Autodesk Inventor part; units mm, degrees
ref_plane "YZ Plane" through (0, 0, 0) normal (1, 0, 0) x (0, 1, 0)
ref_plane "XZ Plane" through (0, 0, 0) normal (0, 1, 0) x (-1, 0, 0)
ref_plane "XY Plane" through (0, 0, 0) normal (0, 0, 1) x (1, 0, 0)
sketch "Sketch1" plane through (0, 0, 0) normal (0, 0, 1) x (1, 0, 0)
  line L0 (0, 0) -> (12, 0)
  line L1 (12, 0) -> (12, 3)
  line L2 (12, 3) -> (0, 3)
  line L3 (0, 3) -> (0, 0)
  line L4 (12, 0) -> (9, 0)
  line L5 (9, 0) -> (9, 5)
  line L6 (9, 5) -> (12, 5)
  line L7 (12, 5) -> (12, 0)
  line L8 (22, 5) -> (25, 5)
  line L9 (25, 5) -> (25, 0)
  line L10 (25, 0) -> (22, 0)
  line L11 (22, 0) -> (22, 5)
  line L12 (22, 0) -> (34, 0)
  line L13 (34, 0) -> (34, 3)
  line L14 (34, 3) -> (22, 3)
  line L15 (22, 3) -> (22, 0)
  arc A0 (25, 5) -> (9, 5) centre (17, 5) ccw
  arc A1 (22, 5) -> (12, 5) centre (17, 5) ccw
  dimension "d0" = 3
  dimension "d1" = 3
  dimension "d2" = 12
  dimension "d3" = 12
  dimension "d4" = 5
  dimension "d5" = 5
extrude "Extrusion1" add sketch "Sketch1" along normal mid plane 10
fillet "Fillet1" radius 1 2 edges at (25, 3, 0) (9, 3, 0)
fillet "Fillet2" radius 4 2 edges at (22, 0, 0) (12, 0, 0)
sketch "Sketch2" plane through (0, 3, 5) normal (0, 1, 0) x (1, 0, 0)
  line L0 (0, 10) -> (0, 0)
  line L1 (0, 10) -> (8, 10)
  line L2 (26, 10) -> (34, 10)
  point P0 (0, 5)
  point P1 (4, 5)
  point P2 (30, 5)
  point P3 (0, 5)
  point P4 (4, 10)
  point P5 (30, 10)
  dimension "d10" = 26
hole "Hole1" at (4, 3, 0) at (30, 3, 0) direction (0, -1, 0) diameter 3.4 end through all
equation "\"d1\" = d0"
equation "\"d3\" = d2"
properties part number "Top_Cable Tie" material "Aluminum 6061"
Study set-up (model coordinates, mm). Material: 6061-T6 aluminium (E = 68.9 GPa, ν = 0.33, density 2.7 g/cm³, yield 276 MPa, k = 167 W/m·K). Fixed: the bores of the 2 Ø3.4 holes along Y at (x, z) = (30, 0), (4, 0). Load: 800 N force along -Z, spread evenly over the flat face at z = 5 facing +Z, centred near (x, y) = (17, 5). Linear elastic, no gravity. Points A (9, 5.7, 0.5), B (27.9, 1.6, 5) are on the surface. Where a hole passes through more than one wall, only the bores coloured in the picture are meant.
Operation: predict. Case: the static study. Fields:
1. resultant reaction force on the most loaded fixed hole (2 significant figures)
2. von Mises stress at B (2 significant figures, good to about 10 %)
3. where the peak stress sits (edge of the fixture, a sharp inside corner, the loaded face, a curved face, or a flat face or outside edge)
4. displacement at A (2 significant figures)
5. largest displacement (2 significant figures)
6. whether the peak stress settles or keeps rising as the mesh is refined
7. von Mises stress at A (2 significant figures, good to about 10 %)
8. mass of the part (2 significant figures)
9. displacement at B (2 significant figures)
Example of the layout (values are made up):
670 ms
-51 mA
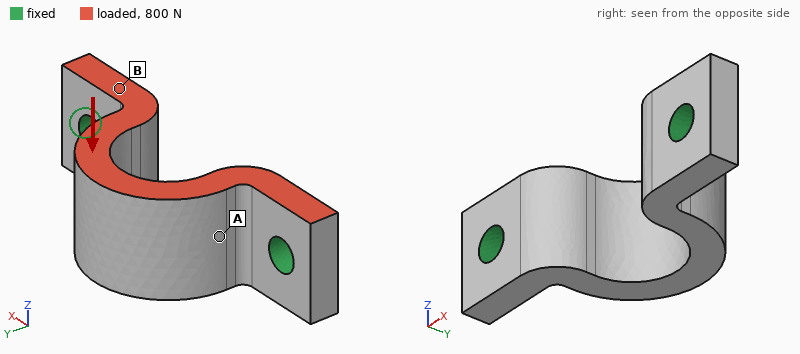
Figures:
400 N
61 MPa
edge of the fixture
18 µm
47 µm
keeps rising
22 MPa
3.6 g
7.3 µm
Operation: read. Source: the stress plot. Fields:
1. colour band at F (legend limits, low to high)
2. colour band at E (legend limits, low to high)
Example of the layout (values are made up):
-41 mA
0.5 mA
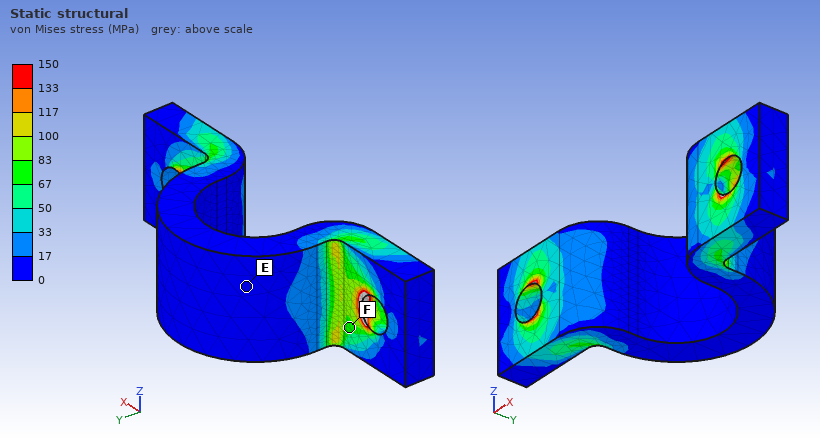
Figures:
67 to 83 MPa
0 to 17 MPa
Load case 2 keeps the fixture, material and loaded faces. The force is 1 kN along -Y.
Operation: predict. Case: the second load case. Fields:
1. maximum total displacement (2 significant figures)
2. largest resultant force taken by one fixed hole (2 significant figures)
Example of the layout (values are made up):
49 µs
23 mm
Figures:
54 µm
520 N
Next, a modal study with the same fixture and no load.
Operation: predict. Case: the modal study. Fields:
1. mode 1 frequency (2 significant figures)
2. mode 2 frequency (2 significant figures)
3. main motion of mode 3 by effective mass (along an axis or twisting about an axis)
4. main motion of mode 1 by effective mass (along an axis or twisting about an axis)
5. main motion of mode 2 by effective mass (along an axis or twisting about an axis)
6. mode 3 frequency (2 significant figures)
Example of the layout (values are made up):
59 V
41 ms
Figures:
13 kHz
26 kHz
along Y
along Z
along X
30 kHz
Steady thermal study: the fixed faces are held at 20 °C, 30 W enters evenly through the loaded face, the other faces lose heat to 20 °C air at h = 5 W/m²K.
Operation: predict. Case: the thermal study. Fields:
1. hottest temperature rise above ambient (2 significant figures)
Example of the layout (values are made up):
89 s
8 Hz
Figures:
27 K
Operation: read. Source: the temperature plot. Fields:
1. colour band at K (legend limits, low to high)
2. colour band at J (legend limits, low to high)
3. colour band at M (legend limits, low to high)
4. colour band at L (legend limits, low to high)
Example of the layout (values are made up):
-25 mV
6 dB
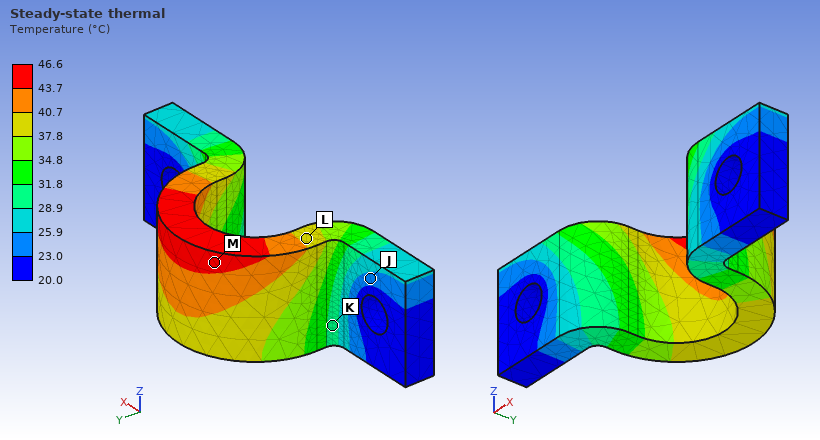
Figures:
28.9 to 31.8 °C
23.0 to 25.9 °C
43.7 to 46.6 °C
37.8 to 40.7 °C
